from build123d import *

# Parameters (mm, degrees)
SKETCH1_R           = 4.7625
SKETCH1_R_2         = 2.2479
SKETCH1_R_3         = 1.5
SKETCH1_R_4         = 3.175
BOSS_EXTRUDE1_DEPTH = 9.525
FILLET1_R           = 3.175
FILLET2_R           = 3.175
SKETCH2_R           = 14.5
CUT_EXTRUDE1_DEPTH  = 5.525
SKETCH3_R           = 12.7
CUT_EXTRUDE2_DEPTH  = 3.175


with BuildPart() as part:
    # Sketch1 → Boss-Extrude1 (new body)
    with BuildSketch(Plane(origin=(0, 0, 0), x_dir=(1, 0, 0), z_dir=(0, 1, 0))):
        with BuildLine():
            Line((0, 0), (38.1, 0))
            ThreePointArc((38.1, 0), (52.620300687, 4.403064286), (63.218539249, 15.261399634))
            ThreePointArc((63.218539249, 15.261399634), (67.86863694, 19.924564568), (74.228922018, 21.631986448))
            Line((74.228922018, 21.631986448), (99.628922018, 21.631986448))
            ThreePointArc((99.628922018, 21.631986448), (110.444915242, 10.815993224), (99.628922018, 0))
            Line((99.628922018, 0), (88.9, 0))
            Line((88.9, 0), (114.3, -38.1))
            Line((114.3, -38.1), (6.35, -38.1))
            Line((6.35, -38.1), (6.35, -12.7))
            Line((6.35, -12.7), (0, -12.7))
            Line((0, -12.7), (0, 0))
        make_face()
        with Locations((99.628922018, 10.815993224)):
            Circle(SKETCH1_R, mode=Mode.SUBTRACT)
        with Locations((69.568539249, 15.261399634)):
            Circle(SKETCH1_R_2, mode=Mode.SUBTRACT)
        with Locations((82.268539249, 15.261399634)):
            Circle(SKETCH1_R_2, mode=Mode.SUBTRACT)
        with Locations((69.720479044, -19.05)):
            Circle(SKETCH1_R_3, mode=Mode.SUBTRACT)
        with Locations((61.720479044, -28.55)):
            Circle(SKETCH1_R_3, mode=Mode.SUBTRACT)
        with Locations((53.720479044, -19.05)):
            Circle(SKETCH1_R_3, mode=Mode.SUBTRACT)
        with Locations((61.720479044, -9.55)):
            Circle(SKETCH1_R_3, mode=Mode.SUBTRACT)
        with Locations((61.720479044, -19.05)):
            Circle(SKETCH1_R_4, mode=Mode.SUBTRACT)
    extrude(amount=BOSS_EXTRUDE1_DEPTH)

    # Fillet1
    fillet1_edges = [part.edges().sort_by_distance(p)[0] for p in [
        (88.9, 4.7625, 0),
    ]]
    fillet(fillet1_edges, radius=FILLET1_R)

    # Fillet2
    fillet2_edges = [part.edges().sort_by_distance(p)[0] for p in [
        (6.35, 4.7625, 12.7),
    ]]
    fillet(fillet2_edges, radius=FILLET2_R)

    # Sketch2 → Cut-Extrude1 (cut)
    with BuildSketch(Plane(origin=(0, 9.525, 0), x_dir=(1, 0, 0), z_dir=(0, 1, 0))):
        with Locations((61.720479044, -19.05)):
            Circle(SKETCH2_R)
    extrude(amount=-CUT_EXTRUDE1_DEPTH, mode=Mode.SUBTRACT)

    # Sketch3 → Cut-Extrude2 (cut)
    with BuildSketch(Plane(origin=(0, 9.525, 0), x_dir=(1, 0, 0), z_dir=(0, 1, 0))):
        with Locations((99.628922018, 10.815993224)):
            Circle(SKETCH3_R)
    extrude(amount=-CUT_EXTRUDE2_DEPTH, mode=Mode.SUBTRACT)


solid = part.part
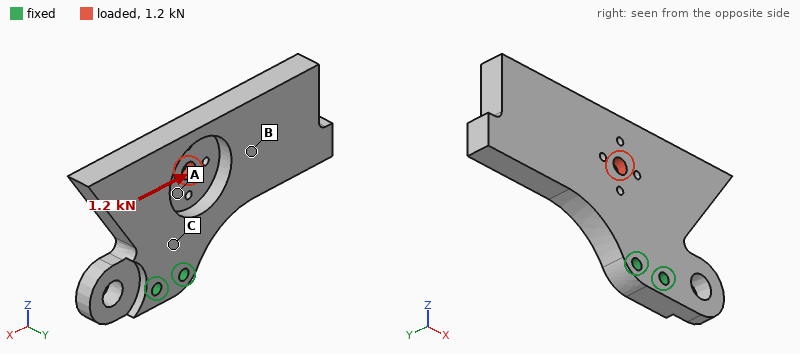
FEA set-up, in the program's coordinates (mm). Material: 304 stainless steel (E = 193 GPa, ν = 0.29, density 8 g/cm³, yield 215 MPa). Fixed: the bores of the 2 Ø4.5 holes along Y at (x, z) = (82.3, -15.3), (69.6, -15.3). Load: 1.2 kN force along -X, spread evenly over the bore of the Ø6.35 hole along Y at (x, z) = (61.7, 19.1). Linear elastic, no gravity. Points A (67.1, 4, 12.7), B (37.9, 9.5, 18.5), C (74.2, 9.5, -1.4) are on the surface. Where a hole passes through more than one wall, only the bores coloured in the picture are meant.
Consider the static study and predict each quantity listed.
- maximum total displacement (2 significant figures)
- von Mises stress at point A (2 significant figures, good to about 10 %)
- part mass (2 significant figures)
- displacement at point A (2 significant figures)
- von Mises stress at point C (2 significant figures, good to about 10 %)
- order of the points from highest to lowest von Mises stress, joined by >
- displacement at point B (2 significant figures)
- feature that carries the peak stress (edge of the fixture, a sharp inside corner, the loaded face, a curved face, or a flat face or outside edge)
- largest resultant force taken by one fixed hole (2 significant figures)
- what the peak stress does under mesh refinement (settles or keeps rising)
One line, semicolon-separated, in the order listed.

23 µm; 17 MPa; 320 g; 7.1 µm; 12 MPa; A > C > B; 12 µm; edge of the fixture; 2.5 kN; keeps rising
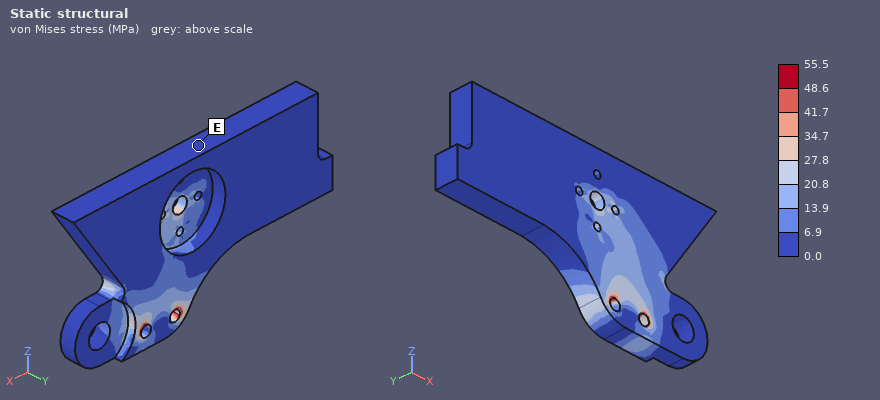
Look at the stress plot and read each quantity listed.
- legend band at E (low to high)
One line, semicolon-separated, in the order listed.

0.0 to 6.9 MPa
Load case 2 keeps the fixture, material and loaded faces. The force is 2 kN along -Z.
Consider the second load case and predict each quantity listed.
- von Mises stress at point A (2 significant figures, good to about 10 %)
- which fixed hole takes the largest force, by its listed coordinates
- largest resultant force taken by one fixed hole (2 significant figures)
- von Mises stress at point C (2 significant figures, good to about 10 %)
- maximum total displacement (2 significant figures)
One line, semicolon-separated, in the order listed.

25 MPa; (69.6, -15.3); 2.8 kN; 10 MPa; 23 µm
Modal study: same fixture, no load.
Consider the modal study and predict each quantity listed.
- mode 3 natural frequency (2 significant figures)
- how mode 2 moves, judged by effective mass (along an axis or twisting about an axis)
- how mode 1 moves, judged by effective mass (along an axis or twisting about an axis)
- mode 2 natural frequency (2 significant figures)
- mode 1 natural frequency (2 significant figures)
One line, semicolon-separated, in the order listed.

2300 Hz; along Y; along Y; 1900 Hz; 970 Hz
